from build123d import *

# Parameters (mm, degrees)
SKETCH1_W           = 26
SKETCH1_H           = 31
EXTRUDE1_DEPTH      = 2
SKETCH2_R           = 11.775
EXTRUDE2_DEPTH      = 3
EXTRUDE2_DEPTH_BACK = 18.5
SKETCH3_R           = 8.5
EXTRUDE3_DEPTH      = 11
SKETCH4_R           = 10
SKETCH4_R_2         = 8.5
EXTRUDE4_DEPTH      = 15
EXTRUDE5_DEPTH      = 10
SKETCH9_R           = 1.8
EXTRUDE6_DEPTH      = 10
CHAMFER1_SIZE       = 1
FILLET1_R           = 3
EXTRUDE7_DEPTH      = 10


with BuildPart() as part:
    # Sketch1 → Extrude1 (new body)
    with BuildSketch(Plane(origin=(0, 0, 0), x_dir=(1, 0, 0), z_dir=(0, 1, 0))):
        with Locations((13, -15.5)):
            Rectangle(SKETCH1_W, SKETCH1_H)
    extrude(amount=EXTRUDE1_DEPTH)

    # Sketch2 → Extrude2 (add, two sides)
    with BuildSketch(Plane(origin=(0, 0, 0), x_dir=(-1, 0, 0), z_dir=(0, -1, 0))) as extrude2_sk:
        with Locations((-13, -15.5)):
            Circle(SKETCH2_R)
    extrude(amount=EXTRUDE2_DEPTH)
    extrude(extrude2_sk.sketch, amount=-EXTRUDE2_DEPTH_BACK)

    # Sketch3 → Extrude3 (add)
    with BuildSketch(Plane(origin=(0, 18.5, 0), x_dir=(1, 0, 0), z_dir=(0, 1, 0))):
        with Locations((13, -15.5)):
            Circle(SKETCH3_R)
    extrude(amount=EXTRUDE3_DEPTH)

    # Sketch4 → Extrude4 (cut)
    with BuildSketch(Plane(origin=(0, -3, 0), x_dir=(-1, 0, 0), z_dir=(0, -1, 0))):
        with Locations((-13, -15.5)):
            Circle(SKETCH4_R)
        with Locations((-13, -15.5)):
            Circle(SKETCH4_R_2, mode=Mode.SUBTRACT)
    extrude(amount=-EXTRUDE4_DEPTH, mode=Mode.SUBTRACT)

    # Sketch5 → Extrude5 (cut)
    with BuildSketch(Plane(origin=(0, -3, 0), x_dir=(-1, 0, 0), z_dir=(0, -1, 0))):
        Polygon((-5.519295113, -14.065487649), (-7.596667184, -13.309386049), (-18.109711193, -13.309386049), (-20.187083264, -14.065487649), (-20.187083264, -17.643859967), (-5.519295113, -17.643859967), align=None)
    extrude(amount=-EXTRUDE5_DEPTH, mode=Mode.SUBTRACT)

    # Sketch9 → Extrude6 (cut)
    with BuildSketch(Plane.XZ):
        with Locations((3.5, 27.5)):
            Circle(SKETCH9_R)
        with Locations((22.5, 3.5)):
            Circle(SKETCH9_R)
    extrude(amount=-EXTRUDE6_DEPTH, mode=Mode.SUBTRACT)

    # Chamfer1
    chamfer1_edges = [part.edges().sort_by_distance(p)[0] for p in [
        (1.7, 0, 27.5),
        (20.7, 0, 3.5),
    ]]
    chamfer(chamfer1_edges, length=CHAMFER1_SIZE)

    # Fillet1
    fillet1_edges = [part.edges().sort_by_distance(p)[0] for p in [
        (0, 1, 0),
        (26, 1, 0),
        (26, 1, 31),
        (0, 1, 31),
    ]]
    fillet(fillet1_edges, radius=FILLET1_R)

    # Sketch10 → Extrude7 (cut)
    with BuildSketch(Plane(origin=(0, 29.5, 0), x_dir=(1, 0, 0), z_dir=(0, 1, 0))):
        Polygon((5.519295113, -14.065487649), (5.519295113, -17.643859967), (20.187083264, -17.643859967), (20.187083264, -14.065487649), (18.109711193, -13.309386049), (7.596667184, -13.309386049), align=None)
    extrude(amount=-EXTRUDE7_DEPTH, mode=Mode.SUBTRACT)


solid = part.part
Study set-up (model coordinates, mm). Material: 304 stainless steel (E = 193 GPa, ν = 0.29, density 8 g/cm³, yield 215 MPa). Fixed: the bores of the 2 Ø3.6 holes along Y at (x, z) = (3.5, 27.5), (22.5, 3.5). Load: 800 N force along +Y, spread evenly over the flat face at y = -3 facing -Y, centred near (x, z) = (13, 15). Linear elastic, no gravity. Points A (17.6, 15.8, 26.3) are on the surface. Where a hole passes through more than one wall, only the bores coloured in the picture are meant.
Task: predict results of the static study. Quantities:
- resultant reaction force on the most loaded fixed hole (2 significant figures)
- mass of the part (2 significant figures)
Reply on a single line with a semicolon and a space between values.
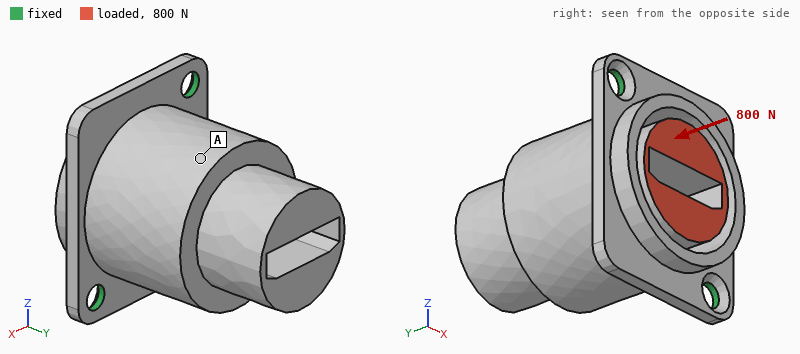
410 N; 80 g
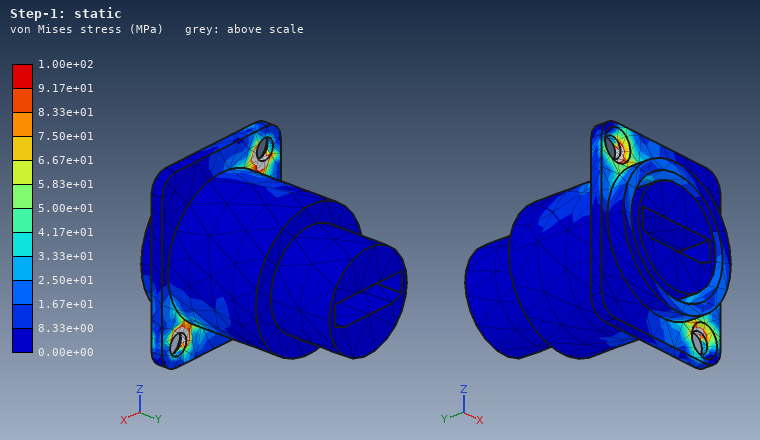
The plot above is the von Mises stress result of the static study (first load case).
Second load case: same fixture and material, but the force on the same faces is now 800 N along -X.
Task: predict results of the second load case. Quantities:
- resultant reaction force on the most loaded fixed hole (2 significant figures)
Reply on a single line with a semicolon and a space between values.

410 N
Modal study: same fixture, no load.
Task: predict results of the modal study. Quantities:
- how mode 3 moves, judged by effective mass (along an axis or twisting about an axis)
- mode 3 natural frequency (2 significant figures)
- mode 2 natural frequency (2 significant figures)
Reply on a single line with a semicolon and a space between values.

along Y; 6900 Hz; 5700 Hz
